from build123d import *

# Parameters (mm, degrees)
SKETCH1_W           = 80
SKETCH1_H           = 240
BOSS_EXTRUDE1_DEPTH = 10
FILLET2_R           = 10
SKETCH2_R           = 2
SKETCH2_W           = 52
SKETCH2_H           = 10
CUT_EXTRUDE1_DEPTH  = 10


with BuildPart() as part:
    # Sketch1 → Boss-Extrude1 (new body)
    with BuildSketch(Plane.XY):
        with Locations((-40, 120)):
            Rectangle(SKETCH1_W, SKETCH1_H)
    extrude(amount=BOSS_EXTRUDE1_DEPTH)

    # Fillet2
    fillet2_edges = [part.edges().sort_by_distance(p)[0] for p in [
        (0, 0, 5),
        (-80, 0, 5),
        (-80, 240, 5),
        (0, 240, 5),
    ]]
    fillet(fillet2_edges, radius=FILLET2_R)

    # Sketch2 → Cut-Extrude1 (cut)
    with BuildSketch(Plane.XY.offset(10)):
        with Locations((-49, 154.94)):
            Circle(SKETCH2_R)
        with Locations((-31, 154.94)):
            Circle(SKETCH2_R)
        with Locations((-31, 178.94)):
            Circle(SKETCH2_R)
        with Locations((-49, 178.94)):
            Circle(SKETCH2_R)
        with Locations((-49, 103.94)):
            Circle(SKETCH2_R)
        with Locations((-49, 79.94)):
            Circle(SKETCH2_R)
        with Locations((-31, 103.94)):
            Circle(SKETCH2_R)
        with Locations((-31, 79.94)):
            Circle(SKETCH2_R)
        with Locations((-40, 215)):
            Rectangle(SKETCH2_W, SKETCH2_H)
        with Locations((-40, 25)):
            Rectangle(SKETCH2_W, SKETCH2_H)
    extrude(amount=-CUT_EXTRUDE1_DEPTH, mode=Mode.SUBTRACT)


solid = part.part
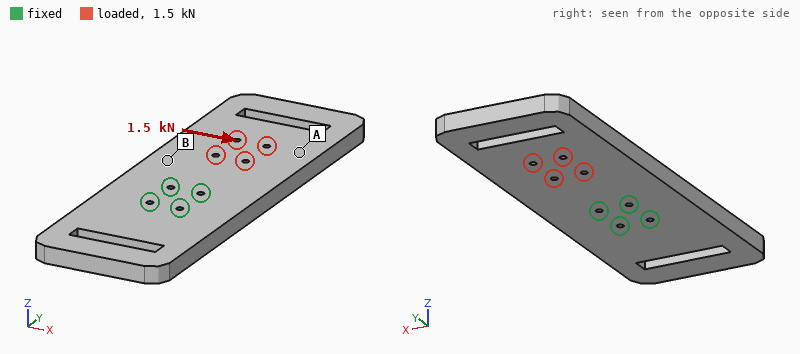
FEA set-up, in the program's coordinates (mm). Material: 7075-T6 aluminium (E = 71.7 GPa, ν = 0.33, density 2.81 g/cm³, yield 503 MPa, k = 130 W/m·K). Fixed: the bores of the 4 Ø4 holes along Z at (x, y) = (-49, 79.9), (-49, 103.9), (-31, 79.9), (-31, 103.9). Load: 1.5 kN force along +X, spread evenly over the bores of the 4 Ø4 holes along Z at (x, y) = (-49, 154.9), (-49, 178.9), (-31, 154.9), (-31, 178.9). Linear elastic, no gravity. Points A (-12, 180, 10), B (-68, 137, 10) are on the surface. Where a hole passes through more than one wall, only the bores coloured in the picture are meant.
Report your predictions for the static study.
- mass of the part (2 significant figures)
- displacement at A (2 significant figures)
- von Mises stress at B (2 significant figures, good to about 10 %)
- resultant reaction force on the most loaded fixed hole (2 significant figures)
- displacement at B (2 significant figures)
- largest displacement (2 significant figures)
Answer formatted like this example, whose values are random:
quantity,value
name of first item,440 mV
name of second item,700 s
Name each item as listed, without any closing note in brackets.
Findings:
quantity,value
mass of the part,510 g
displacement at A,24 µm
von Mises stress at B,3.9 MPa
resultant reaction force on the most loaded fixed hole,2.2 kN
displacement at B,12 µm
largest displacement,39 µm
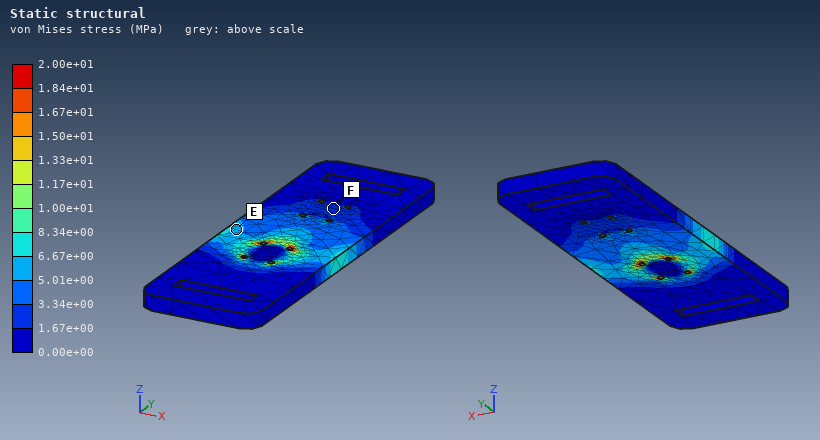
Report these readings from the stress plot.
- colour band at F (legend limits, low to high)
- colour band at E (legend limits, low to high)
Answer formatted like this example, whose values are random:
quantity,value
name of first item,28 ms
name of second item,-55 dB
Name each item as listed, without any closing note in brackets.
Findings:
quantity,value
colour band at F,1.67e+00 to 3.34e+00 MPa
colour band at E,5.01e+00 to 6.67e+00 MPa
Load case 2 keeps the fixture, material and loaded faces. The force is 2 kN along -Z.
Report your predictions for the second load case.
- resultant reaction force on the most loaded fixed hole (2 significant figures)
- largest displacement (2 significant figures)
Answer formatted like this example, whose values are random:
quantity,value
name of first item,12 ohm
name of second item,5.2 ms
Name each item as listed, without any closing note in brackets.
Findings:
quantity,value
resultant reaction force on the most loaded fixed hole,2.2 kN
largest displacement,1.1 mm
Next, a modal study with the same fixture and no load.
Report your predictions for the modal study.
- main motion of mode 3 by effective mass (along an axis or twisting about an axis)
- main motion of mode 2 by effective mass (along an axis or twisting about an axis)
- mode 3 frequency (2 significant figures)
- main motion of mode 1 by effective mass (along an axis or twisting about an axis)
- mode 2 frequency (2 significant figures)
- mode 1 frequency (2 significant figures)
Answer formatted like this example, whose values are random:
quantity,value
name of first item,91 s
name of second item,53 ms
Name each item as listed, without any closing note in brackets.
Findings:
quantity,value
main motion of mode 3 by effective mass,twisting about Y
main motion of mode 2 by effective mass,along Z
mode 3 frequency,1400 Hz
main motion of mode 1 by effective mass,along Z
mode 2 frequency,1200 Hz
mode 1 frequency,450 Hz
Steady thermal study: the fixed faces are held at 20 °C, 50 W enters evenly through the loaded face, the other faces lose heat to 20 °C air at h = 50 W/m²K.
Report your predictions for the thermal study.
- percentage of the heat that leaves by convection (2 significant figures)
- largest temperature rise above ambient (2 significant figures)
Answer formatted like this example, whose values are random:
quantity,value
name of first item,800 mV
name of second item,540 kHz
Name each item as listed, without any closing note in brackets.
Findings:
quantity,value
percentage of the heat that leaves by convection,40 %
largest temperature rise above ambient,24 K
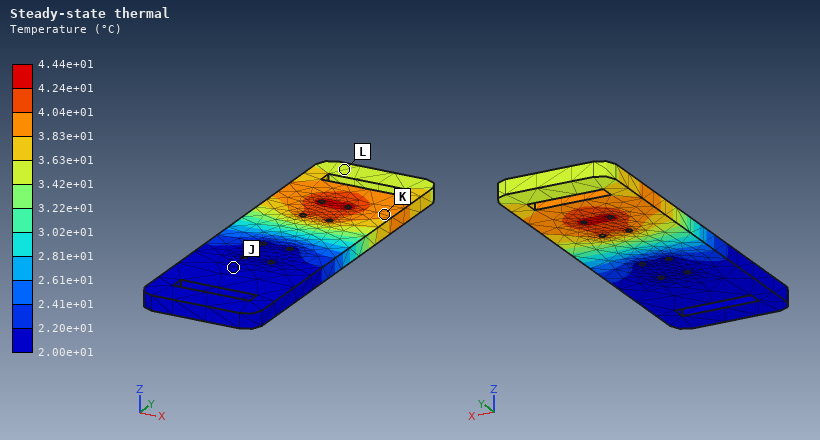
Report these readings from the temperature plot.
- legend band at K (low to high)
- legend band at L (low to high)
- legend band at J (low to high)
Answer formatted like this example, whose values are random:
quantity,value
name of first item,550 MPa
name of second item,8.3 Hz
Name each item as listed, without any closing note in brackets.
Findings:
quantity,value
legend band at K,3.83e+01 to 4.04e+01 °C
legend band at L,3.42e+01 to 3.63e+01 °C
legend band at J,2.00e+01 to 2.20e+01 °C
